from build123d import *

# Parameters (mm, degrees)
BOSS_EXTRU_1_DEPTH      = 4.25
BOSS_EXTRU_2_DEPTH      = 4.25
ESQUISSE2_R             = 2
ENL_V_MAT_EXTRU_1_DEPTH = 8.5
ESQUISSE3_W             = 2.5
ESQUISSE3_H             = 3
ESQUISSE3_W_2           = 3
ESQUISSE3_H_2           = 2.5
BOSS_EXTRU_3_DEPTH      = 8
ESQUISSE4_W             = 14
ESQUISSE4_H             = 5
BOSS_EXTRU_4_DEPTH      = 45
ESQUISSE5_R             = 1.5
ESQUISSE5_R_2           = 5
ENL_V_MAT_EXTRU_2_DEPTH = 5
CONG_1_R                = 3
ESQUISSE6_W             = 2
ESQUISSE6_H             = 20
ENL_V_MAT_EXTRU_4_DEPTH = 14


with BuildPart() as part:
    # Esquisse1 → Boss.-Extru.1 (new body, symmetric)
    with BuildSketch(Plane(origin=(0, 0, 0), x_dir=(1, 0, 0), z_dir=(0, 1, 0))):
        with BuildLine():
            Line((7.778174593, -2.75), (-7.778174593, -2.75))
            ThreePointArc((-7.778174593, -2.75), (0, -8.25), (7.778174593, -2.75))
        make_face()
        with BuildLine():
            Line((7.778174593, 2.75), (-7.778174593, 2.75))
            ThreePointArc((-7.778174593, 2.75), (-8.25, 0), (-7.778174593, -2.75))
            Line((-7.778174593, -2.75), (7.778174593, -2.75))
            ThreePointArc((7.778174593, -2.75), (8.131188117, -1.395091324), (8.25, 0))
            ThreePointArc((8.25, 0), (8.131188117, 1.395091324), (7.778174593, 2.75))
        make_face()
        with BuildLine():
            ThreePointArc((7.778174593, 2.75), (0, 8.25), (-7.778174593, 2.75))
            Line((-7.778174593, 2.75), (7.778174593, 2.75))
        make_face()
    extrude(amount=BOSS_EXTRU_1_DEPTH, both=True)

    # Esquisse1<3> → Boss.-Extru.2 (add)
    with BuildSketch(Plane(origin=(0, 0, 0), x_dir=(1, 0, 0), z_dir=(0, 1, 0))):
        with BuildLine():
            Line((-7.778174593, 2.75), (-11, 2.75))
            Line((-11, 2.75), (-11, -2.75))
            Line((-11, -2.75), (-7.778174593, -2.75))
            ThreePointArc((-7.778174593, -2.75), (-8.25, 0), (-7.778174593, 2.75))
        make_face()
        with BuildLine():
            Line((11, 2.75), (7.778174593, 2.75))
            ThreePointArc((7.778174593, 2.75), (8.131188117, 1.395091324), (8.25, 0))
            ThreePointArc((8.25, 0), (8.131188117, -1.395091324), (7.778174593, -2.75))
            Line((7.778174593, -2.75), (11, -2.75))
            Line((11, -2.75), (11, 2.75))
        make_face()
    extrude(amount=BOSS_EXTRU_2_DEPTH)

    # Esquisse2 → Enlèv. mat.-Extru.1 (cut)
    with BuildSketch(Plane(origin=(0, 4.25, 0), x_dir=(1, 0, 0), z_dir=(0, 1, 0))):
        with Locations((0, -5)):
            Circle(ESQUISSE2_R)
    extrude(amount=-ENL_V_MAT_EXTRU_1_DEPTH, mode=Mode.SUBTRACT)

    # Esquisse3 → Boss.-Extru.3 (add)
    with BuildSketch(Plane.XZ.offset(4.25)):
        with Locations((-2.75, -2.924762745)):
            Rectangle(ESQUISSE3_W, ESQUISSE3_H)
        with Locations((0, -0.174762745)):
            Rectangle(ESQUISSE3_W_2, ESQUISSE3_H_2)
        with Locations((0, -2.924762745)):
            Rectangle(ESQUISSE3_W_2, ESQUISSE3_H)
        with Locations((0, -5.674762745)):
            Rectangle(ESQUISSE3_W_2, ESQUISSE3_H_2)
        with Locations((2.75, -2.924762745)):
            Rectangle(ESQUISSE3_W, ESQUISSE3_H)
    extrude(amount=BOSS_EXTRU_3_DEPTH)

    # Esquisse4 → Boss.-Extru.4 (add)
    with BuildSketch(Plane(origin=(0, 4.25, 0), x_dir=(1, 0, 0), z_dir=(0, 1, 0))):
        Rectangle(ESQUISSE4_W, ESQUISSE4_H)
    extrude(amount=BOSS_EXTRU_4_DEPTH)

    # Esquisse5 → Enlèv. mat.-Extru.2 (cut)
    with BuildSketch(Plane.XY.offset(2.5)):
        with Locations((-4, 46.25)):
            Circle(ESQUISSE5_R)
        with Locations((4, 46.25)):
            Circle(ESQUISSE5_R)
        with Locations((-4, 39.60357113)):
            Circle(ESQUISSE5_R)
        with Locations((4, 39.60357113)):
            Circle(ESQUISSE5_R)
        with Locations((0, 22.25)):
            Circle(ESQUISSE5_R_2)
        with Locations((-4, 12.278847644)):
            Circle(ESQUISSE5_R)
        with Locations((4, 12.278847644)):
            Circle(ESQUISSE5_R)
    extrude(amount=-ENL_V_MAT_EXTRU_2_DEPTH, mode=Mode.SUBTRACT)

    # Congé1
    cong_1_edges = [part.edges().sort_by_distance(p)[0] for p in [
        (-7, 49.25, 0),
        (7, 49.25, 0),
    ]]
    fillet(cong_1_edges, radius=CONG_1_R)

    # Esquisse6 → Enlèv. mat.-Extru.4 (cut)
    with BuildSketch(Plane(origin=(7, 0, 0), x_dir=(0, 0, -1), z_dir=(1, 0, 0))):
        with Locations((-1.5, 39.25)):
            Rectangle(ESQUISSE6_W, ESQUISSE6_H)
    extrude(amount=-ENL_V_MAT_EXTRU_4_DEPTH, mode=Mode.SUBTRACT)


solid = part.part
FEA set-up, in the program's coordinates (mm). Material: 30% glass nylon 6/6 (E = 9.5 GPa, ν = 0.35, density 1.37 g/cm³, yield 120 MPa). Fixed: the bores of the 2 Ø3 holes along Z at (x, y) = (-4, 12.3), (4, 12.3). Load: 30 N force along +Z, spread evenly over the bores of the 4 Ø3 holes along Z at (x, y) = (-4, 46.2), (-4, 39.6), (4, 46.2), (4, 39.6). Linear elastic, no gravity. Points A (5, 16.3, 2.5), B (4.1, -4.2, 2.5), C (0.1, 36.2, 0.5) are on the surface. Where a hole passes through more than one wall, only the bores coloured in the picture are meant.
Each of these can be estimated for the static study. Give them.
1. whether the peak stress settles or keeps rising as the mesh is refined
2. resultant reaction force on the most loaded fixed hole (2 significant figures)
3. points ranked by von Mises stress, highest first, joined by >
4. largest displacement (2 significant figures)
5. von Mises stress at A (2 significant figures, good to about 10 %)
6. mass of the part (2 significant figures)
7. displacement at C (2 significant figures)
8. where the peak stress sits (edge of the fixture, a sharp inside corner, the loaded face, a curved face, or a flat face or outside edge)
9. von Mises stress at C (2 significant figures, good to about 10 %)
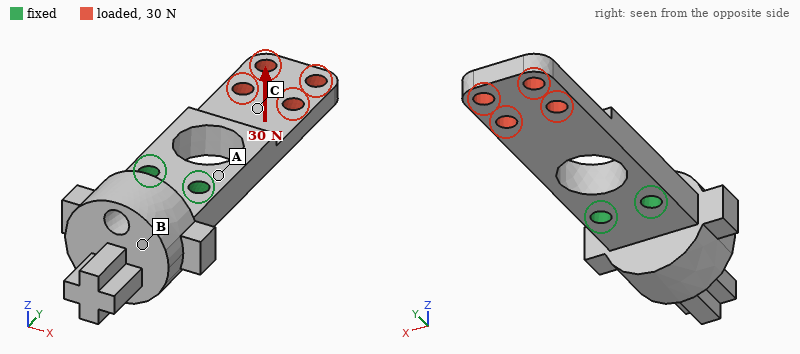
keeps rising
15 N
A > C > B
0.69 mm
23 MPa
5.7 g
0.31 mm
a sharp inside corner
11 MPa
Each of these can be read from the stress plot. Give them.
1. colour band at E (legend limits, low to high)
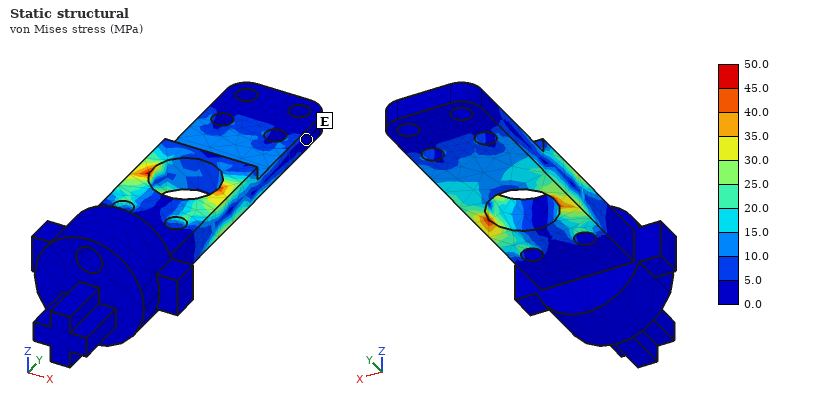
0.0 to 5.0 MPa
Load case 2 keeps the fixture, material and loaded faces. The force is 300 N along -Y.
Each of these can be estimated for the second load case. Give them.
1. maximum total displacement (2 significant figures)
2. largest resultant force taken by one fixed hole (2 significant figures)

0.23 mm
150 N
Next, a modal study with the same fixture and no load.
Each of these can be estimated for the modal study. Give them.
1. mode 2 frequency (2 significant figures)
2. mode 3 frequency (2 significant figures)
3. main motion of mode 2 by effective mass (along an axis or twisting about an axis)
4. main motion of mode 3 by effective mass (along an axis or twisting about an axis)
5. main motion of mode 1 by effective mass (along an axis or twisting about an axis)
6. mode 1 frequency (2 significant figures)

3600 Hz
3800 Hz
along Z
along X
along Z
1400 Hz
